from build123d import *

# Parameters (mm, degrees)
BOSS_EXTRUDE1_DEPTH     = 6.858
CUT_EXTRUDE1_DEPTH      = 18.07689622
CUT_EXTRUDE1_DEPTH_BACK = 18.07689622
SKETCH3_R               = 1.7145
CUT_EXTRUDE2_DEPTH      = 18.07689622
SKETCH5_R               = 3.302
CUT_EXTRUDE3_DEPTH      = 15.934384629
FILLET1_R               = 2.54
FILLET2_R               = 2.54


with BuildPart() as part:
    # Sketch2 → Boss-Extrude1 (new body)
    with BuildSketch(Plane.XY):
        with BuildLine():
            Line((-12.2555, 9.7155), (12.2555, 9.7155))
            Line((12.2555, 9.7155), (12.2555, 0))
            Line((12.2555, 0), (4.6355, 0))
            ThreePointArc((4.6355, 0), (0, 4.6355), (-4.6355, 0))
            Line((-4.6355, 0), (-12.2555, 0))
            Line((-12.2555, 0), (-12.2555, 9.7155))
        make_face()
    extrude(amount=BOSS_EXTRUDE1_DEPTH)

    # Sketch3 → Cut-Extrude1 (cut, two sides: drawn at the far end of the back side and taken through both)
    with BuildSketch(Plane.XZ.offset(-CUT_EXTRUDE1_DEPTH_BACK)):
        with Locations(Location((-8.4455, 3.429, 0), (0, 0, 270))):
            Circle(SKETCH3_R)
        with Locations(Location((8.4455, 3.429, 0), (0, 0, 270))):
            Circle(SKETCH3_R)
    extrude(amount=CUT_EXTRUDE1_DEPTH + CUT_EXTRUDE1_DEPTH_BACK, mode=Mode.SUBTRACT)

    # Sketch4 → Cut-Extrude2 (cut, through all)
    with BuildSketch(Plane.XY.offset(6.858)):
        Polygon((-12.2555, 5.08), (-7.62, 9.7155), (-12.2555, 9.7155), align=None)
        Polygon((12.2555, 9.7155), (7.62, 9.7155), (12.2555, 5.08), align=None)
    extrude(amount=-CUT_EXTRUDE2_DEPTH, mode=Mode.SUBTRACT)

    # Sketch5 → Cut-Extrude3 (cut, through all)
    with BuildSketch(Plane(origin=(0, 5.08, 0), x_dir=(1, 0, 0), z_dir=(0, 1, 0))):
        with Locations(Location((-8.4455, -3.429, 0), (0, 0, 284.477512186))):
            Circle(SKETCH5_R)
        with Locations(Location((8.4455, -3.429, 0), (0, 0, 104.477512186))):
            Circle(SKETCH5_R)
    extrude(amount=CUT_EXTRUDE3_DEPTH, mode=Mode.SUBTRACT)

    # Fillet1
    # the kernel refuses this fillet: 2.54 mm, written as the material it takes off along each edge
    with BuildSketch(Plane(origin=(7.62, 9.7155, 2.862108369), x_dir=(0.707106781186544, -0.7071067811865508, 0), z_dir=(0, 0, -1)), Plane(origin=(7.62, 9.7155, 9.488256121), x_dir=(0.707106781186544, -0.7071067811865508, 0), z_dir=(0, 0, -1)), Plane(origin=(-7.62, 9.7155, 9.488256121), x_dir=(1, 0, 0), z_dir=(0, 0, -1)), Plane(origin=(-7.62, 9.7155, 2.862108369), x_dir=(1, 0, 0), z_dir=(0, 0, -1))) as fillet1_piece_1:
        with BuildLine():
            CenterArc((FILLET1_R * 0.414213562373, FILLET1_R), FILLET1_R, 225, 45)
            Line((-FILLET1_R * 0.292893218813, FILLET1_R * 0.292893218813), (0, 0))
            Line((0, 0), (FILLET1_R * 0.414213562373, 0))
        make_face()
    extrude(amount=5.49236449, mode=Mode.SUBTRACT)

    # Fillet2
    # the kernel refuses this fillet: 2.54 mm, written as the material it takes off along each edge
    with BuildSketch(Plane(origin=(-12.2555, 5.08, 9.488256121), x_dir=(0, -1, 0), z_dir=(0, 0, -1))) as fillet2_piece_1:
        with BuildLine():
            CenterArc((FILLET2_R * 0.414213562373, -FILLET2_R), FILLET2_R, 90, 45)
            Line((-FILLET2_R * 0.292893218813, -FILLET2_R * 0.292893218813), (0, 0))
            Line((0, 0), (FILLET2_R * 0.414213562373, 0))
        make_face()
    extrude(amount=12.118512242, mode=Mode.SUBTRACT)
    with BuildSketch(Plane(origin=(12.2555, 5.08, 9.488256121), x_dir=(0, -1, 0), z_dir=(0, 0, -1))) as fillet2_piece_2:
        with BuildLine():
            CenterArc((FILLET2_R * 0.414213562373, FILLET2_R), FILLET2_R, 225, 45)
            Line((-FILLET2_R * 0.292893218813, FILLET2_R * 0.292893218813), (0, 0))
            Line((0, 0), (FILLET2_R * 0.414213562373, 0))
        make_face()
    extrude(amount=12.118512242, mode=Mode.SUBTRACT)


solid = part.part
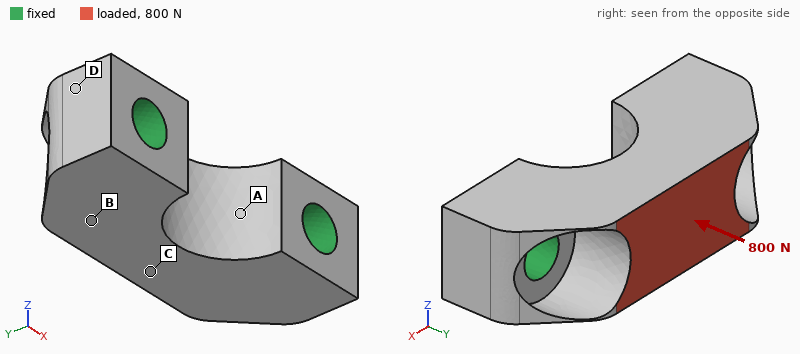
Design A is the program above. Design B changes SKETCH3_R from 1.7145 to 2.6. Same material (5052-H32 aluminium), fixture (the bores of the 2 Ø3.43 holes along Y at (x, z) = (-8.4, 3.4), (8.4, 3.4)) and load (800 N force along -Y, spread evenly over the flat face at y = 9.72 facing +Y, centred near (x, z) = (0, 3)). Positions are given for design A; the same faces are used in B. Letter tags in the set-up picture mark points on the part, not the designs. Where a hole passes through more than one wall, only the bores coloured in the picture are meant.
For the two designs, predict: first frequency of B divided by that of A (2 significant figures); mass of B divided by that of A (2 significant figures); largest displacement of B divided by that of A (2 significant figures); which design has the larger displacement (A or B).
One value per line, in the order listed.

1.2
0.87
0.79
A
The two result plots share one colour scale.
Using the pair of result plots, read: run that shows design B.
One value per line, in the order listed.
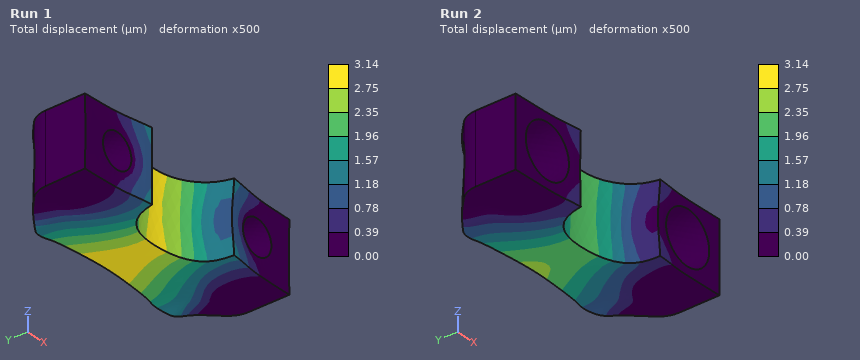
Run 2
